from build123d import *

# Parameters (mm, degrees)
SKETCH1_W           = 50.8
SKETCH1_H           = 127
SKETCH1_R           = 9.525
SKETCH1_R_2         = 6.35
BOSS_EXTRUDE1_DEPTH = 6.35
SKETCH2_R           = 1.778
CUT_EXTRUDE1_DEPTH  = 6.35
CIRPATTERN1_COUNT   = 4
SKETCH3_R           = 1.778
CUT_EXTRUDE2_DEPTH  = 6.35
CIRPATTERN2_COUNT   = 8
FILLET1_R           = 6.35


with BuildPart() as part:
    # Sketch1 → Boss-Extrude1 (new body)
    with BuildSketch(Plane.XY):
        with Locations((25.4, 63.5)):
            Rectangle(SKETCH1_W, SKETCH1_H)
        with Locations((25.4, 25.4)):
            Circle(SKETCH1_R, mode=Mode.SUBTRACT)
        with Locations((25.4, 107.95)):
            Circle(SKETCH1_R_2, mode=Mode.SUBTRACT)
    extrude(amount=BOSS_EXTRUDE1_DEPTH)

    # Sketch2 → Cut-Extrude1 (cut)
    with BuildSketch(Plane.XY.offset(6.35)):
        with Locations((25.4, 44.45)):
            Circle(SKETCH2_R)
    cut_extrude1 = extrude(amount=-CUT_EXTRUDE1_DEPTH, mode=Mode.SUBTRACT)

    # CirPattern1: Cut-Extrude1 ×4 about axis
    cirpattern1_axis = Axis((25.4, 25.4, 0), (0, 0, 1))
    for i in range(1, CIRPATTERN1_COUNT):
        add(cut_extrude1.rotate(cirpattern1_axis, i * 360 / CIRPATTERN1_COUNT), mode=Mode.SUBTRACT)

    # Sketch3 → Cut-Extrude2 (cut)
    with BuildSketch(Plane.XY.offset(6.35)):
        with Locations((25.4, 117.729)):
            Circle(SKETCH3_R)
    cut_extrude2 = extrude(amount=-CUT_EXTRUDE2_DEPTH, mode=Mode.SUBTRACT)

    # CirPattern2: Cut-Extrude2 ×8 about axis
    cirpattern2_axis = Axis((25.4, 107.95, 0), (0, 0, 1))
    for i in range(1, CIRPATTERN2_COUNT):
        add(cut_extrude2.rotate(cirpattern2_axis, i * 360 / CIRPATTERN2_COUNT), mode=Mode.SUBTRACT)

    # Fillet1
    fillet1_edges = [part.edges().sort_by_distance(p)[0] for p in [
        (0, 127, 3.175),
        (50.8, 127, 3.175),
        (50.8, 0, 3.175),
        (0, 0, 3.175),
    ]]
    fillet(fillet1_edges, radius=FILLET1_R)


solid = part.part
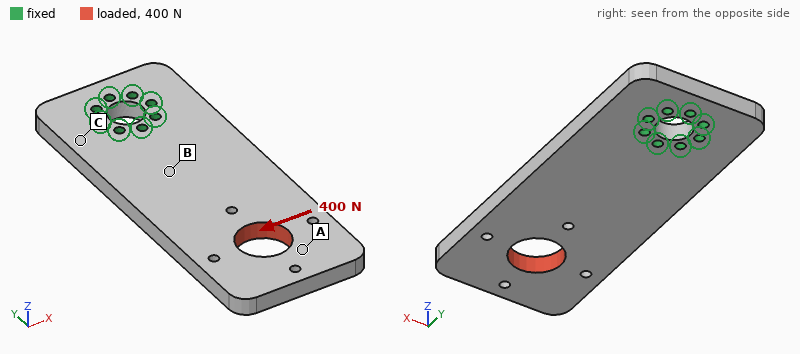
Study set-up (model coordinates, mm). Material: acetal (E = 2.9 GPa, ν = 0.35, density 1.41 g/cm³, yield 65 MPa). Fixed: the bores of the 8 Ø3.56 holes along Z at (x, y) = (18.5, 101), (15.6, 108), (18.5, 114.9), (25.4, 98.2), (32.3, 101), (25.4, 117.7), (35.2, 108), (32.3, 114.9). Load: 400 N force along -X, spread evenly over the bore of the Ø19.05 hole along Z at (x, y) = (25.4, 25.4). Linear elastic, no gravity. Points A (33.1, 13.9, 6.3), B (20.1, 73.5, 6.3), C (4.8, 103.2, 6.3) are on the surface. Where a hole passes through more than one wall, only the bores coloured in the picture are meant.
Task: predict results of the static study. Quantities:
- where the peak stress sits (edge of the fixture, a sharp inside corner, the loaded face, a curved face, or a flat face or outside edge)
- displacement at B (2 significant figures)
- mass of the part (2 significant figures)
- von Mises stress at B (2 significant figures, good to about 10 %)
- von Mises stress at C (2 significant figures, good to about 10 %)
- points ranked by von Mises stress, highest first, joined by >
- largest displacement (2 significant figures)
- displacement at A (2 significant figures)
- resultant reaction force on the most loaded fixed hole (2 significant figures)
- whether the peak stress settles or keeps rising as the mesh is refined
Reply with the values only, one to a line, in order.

edge of the fixture
0.17 mm
53 g
3.5 MPa
6.3 MPa
C > B > A
0.87 mm
0.74 mm
510 N
keeps rising
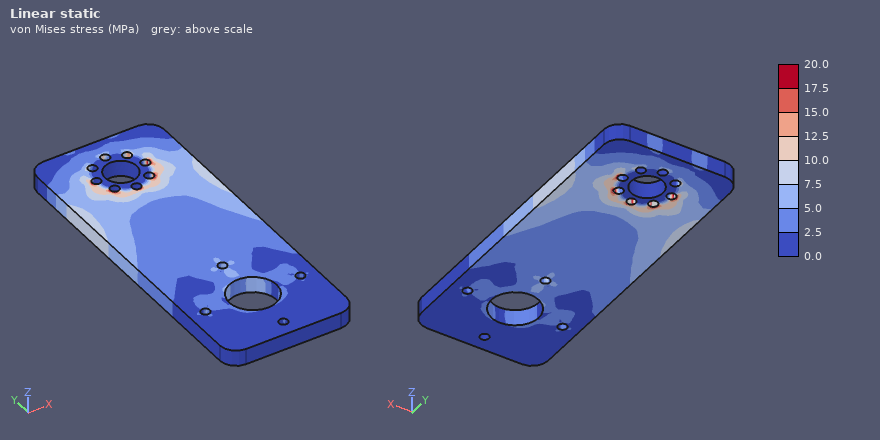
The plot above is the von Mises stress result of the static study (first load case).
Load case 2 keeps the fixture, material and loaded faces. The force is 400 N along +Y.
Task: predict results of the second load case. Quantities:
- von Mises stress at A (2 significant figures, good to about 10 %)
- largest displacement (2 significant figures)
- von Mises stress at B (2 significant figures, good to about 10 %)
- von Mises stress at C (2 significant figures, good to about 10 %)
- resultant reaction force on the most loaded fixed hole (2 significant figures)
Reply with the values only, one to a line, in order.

1.1 MPa
50 µm
1.4 MPa
0.61 MPa
93 N
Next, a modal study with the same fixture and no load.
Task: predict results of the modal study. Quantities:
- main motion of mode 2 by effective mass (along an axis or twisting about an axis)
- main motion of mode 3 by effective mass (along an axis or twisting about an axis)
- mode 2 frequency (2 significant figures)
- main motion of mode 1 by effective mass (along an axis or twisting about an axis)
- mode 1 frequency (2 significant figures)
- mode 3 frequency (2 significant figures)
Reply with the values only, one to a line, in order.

twisting about Y
along X
550 Hz
along Z
160 Hz
820 Hz
